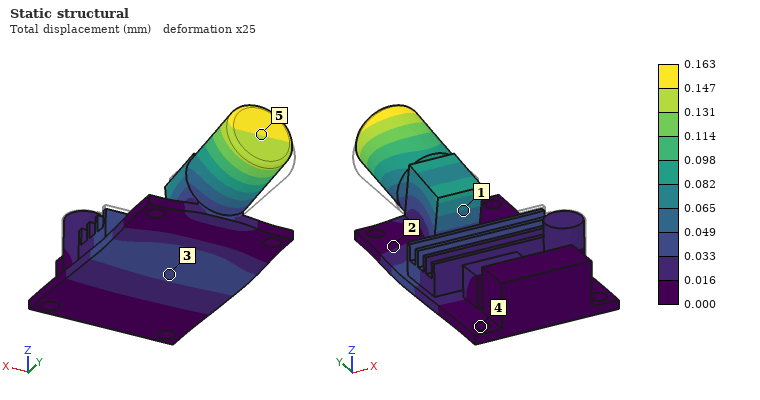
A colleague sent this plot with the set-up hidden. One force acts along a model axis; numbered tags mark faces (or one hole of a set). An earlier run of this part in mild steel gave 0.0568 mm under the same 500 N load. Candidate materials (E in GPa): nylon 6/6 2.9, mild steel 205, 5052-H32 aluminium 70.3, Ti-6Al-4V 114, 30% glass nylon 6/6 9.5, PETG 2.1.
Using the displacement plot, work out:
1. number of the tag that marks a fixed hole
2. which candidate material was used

4
5052-H32 aluminium
